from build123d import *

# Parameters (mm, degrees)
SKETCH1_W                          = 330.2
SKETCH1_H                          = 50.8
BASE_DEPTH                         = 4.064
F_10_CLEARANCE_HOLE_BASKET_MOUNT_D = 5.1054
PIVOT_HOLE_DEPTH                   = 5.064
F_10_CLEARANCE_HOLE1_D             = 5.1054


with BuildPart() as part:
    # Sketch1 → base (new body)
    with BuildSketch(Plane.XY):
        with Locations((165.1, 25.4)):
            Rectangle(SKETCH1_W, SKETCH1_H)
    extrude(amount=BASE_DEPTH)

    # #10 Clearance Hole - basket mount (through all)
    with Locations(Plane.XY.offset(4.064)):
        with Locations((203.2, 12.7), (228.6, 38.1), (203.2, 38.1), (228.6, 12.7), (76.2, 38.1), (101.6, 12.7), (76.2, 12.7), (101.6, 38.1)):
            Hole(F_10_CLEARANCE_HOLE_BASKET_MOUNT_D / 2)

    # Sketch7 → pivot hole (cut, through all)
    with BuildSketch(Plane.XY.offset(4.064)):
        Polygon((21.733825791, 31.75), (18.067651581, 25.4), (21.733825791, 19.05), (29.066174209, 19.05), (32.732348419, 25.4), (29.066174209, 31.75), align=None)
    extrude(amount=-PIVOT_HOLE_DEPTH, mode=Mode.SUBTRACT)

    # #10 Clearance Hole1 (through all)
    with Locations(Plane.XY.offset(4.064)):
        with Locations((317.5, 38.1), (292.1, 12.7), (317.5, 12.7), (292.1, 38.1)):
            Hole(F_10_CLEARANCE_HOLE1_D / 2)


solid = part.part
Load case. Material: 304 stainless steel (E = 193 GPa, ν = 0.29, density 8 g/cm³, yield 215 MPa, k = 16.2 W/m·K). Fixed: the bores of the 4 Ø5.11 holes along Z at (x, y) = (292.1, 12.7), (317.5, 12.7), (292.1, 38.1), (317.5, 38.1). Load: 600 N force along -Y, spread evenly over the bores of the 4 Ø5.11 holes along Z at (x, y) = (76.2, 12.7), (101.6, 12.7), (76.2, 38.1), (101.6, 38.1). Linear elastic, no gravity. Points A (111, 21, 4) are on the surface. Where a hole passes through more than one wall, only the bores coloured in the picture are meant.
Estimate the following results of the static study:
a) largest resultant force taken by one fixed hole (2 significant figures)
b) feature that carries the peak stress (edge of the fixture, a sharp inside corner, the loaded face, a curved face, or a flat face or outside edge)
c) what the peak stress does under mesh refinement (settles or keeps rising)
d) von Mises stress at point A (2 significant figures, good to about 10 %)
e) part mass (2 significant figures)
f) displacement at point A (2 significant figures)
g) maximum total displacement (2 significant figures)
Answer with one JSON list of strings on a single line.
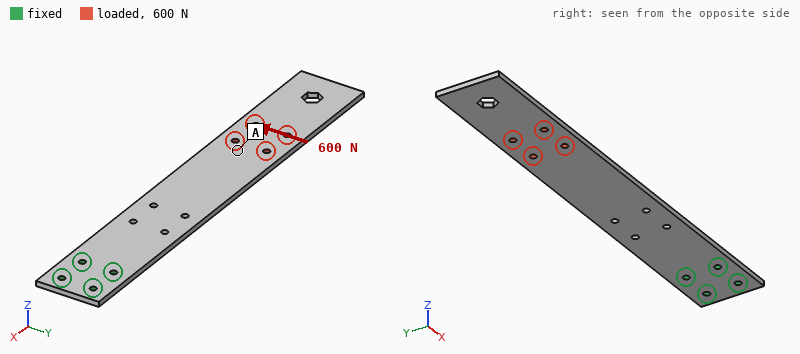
["3.2 kN", "edge of the fixture", "keeps rising", "7.2 MPa", "530 g", "0.19 mm", "0.37 mm"]
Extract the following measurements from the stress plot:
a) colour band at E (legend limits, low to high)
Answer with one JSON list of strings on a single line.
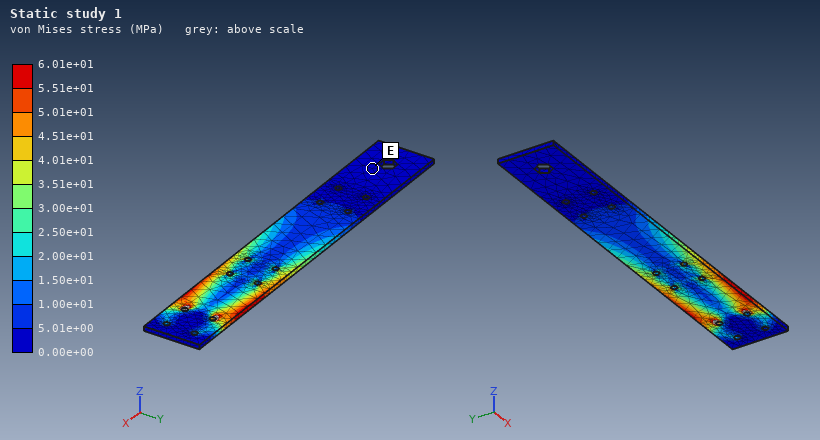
["0.00e+00 to 5.01e+00 MPa"]
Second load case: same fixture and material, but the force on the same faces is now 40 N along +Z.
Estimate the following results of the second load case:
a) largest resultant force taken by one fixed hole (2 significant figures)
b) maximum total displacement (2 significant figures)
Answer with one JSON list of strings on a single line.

["52 N", "3.4 mm"]
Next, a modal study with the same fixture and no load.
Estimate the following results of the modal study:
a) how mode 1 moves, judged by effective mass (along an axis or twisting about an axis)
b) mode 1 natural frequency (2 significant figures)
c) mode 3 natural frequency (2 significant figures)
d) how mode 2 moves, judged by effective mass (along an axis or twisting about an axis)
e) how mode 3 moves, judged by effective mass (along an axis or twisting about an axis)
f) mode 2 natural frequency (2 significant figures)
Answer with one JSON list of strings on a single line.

["along Z", "38 Hz", "420 Hz", "along Z", "twisting about X", "240 Hz"]
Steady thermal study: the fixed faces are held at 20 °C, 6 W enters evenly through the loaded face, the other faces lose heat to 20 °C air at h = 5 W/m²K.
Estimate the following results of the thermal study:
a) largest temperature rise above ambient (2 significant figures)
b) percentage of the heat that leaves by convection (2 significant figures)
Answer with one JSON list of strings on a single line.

["72 K", "92 %"]
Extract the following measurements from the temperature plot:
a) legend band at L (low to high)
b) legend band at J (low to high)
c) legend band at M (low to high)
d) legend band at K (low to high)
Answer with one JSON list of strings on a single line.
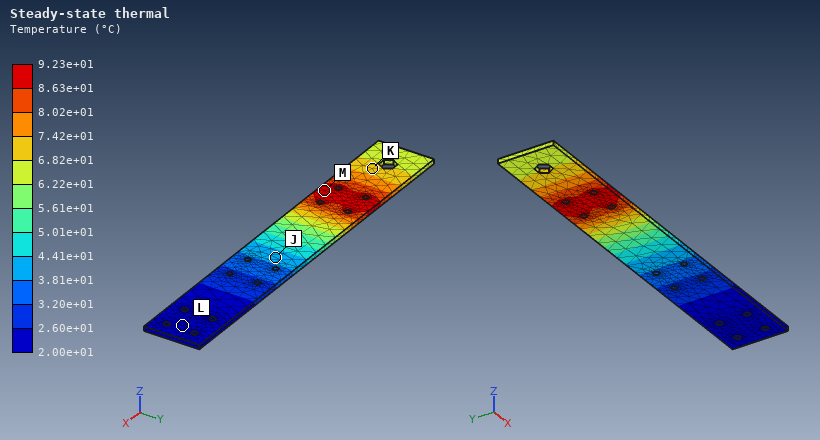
["2.00e+01 to 2.60e+01 °C", "3.81e+01 to 4.41e+01 °C", "8.63e+01 to 9.23e+01 °C", "6.82e+01 to 7.42e+01 °C"]
